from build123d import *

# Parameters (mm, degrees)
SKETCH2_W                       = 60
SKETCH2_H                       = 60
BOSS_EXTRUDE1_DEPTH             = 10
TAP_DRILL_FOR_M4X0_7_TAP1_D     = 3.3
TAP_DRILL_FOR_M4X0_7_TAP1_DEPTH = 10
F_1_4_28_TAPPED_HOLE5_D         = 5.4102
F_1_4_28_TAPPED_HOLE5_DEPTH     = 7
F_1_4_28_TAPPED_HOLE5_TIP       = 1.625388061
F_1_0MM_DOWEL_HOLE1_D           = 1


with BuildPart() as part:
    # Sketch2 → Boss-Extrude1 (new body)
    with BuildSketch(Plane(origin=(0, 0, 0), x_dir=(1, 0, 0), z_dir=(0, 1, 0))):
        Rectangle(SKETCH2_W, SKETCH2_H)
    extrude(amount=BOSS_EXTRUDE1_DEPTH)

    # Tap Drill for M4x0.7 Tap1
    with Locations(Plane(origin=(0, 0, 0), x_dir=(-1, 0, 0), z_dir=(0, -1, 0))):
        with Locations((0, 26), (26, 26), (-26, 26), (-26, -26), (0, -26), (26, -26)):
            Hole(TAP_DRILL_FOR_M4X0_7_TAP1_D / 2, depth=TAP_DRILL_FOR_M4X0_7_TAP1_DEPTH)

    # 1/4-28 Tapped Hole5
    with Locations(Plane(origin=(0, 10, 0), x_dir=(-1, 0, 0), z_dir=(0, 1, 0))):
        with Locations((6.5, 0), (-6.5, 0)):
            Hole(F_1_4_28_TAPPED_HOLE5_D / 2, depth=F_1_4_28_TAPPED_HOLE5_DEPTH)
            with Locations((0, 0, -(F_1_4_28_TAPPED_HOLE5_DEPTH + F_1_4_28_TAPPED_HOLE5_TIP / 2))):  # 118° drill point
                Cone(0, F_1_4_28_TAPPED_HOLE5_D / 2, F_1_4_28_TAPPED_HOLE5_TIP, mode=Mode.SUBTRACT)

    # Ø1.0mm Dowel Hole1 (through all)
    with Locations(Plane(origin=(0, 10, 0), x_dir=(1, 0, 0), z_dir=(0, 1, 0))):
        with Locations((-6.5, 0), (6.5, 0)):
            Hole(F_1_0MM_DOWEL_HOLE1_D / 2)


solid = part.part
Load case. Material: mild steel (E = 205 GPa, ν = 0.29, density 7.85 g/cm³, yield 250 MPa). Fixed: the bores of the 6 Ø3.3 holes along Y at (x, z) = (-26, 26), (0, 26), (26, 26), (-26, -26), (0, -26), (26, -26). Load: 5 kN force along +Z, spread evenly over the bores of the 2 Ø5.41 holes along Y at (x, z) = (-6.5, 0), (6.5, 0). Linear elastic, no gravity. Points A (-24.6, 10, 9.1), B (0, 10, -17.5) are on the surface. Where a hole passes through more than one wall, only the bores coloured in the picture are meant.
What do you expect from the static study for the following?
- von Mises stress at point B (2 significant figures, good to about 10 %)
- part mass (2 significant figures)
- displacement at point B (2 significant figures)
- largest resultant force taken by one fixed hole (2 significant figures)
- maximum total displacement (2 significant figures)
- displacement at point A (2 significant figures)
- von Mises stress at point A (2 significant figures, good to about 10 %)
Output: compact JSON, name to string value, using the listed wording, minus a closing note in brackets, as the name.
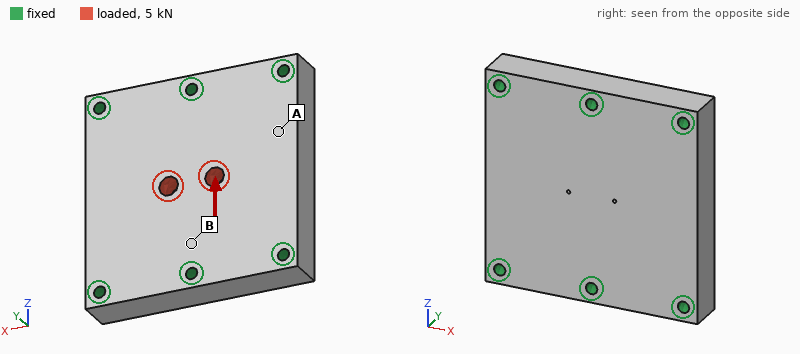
{"von Mises stress at point B": "11 MPa", "part mass": "280 g", "displacement at point B": "0.44 µm", "largest resultant force taken by one fixed hole": "1.3 kN", "maximum total displacement": "1.5 µm", "displacement at point A": "0.31 µm", "von Mises stress at point A": "2.5 MPa"}
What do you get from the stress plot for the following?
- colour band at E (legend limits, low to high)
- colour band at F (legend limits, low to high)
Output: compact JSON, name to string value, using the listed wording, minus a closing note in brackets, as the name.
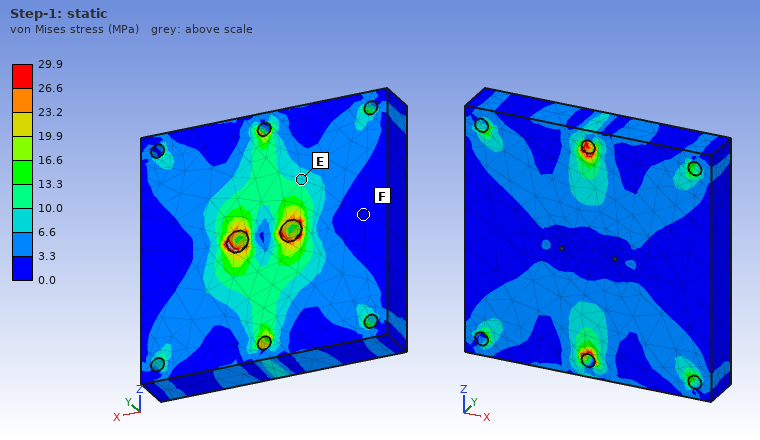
{"colour band at E": "6.6 to 10.0 MPa", "colour band at F": "0.0 to 3.3 MPa"}
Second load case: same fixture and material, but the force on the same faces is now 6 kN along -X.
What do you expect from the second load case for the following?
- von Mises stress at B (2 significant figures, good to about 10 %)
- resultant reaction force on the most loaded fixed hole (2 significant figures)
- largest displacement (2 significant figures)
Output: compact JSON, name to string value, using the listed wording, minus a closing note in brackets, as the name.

{"von Mises stress at B": "10.0 MPa", "resultant reaction force on the most loaded fixed hole": "1.3 kN", "largest displacement": "3.1 µm"}
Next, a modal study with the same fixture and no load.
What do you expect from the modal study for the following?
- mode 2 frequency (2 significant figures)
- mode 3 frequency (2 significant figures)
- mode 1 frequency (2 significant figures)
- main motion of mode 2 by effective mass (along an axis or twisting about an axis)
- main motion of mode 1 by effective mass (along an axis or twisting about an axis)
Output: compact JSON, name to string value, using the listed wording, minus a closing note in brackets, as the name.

{"mode 2 frequency": "17 kHz", "mode 3 frequency": "25 kHz", "mode 1 frequency": "14 kHz", "main motion of mode 2 by effective mass": "twisting about Z", "main motion of mode 1 by effective mass": "along Y"}
